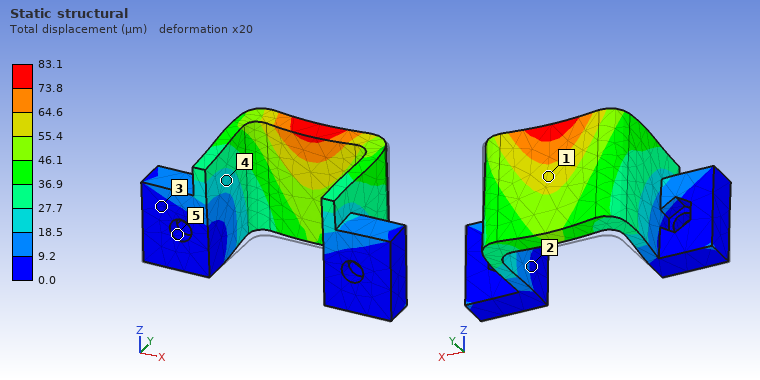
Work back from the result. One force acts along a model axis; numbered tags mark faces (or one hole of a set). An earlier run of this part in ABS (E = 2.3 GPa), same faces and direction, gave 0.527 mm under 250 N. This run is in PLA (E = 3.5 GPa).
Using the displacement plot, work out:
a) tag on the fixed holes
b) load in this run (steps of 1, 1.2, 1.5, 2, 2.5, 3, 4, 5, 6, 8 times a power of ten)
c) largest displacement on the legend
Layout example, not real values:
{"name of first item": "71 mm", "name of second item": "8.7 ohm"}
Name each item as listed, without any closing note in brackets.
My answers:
{"tag on the fixed holes": "5", "load in this run": "60 N", "largest displacement on the legend": "83.1 µm"}
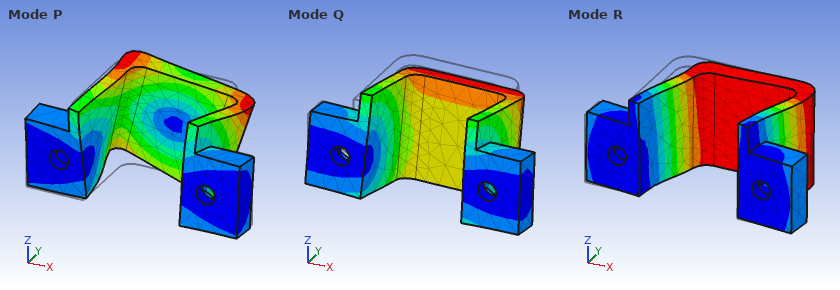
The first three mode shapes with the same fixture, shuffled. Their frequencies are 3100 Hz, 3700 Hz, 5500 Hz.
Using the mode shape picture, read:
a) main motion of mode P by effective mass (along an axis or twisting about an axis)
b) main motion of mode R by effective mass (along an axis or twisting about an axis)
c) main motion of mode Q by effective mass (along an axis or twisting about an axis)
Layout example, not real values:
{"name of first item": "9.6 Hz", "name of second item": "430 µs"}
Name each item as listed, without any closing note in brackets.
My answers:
{"main motion of mode P by effective mass": "twisting about Y", "main motion of mode R by effective mass": "along X", "main motion of mode Q by effective mass": "along Z"}
